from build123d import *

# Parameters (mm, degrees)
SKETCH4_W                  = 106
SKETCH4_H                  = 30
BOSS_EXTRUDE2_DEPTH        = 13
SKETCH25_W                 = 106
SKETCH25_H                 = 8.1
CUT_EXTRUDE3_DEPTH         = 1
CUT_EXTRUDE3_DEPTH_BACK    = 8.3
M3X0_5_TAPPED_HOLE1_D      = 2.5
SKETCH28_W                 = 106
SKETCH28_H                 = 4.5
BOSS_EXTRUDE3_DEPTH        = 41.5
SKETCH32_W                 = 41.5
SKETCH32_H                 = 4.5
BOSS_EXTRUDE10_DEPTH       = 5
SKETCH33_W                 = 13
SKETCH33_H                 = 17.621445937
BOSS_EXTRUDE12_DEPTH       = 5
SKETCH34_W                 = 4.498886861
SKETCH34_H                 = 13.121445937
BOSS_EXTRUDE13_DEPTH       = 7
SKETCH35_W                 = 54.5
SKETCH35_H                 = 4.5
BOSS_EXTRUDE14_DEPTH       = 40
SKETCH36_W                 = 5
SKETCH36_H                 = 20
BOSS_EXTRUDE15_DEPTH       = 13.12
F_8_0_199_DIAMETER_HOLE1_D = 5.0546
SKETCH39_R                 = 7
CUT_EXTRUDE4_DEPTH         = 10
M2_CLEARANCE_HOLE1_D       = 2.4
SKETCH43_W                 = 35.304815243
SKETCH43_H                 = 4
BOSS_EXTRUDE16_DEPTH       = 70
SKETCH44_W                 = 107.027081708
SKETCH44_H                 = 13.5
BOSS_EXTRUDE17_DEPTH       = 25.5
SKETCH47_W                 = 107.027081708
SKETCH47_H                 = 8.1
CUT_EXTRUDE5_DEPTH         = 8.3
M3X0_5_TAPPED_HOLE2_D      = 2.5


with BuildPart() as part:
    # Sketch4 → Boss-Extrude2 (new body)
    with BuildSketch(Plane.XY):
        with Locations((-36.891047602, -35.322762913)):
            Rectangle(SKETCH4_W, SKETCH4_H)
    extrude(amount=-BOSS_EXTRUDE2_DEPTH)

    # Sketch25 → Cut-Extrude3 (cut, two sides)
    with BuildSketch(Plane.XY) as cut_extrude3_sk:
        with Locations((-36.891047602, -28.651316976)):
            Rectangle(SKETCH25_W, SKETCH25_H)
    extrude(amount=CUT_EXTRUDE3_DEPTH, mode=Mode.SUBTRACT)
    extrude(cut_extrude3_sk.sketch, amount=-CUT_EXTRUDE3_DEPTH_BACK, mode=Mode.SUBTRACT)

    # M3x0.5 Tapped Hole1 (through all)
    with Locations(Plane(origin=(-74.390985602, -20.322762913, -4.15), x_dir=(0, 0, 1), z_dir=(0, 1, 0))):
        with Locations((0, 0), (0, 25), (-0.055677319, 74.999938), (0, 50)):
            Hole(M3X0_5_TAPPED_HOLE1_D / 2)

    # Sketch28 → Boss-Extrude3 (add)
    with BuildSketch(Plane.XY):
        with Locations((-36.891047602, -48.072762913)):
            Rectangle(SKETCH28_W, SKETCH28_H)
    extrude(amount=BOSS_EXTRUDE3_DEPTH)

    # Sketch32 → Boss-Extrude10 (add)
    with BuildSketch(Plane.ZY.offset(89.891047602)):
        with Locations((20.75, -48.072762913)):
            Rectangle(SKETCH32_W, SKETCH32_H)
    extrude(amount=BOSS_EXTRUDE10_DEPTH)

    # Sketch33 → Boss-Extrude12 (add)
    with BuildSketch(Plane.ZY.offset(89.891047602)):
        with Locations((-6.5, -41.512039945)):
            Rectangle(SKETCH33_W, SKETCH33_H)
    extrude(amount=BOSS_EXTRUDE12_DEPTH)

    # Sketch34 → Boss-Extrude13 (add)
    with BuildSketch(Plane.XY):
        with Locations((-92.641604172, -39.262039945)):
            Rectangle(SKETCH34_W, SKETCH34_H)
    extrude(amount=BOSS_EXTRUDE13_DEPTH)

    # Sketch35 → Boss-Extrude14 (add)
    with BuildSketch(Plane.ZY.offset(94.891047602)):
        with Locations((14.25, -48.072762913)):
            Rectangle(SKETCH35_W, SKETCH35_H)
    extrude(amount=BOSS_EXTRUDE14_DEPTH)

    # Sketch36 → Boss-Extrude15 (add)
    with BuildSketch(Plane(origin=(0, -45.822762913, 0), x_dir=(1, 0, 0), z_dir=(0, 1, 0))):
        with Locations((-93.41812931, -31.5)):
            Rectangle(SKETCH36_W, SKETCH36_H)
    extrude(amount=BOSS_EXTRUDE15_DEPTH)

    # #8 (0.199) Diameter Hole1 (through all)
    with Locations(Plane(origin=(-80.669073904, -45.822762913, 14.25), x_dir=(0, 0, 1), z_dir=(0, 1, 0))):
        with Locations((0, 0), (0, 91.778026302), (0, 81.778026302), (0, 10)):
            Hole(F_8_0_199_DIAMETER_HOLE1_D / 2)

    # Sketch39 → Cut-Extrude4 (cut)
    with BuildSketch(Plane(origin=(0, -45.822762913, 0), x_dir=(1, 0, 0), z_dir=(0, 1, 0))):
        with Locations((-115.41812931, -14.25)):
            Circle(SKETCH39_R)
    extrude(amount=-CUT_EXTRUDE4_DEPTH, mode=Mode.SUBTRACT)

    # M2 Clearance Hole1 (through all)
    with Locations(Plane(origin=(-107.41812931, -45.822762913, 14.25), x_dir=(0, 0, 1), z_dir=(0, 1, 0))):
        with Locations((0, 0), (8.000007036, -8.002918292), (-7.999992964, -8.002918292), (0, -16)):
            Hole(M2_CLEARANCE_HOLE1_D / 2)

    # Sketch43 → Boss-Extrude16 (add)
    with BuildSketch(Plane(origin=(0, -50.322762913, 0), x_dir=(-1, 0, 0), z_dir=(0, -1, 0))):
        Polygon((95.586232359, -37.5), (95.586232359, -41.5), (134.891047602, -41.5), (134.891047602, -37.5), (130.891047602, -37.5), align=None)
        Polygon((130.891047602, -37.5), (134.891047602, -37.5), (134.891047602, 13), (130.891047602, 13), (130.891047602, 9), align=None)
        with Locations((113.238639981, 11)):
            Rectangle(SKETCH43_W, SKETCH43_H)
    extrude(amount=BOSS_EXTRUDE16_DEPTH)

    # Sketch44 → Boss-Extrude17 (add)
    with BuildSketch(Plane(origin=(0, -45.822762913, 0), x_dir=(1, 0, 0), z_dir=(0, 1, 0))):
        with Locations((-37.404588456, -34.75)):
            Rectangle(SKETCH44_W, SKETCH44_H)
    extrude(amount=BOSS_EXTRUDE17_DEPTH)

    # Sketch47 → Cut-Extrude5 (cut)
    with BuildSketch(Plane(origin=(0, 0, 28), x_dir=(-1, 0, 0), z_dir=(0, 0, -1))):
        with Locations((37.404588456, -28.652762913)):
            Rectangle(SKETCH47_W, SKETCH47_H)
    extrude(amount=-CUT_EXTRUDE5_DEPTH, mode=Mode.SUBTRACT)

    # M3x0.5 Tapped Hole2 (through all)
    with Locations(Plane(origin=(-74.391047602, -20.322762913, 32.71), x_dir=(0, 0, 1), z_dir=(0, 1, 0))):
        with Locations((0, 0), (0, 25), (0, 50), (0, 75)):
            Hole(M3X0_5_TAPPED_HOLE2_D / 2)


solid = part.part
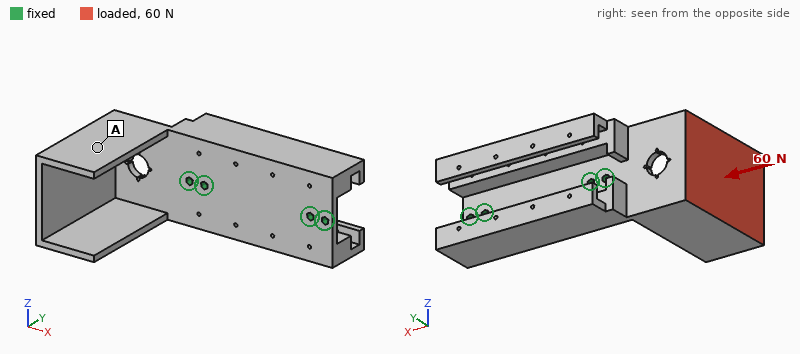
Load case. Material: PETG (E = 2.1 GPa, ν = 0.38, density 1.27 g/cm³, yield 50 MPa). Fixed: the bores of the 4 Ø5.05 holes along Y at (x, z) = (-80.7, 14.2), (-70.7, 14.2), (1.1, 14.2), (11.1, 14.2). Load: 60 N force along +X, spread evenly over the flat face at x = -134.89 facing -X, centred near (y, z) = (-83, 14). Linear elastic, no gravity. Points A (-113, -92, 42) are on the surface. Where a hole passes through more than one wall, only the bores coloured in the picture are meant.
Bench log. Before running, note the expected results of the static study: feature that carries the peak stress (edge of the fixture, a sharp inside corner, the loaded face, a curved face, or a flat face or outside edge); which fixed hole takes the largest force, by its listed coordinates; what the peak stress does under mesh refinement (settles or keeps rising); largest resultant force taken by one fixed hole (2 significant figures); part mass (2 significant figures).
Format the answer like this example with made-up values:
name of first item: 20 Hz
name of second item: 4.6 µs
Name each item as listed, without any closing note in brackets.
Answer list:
feature that carries the peak stress: a sharp inside corner
which fixed hole takes the largest force, by its listed coordinates: (-80.7, 14.2)
what the peak stress does under mesh refinement: keeps rising
largest resultant force taken by one fixed hole: 58 N
part mass: 170 g
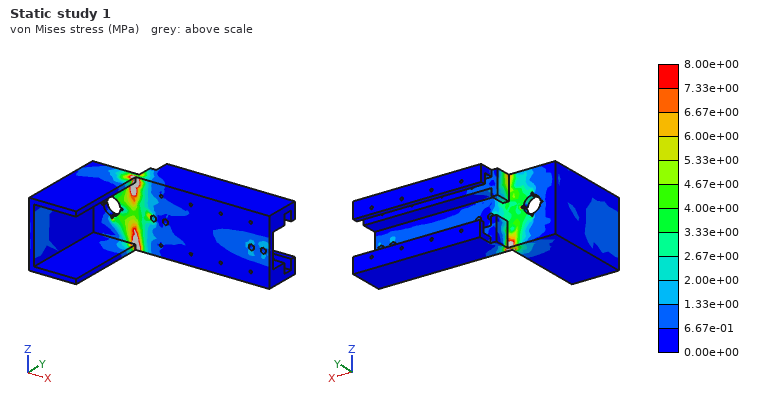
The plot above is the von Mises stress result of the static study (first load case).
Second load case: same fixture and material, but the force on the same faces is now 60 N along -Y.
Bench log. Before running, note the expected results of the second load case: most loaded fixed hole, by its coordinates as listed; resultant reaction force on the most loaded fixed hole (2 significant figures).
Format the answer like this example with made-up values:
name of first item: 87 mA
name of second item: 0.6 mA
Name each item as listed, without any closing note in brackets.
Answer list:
most loaded fixed hole, by its coordinates as listed: (-80.7, 14.2)
resultant reaction force on the most loaded fixed hole: 81 N
